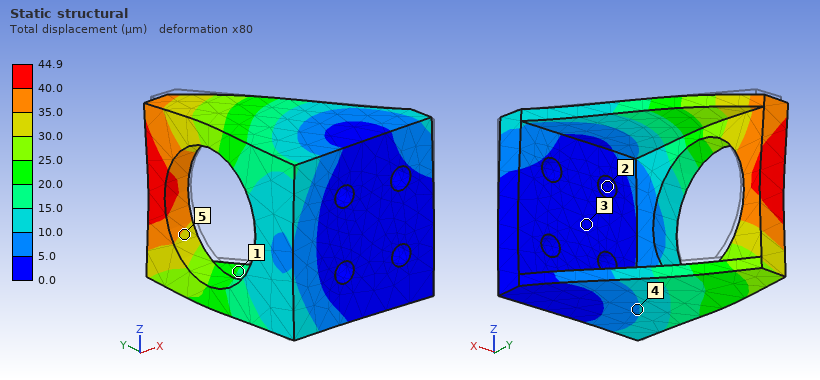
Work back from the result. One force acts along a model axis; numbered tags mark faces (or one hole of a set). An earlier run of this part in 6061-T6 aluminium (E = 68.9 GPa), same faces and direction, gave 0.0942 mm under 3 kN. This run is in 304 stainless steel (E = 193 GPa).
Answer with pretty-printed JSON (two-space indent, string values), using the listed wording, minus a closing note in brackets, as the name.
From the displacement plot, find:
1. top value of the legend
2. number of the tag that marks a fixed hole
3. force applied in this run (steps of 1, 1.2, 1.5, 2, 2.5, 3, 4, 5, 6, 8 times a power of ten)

{
  "top value of the legend": "44.9 µm",
  "number of the tag that marks a fixed hole": "2",
  "force applied in this run": "4 kN"
}
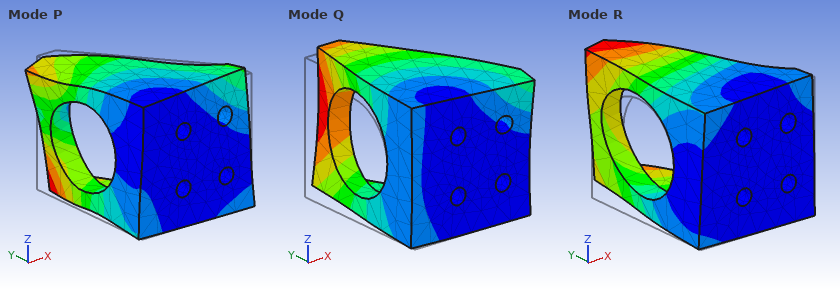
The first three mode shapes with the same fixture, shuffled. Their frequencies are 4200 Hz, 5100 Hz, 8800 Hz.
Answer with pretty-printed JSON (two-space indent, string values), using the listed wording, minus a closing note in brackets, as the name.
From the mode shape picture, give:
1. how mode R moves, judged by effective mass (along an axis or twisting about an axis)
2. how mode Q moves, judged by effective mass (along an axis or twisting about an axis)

{
  "how mode R moves, judged by effective mass": "along Z",
  "how mode Q moves, judged by effective mass": "along X"
}
